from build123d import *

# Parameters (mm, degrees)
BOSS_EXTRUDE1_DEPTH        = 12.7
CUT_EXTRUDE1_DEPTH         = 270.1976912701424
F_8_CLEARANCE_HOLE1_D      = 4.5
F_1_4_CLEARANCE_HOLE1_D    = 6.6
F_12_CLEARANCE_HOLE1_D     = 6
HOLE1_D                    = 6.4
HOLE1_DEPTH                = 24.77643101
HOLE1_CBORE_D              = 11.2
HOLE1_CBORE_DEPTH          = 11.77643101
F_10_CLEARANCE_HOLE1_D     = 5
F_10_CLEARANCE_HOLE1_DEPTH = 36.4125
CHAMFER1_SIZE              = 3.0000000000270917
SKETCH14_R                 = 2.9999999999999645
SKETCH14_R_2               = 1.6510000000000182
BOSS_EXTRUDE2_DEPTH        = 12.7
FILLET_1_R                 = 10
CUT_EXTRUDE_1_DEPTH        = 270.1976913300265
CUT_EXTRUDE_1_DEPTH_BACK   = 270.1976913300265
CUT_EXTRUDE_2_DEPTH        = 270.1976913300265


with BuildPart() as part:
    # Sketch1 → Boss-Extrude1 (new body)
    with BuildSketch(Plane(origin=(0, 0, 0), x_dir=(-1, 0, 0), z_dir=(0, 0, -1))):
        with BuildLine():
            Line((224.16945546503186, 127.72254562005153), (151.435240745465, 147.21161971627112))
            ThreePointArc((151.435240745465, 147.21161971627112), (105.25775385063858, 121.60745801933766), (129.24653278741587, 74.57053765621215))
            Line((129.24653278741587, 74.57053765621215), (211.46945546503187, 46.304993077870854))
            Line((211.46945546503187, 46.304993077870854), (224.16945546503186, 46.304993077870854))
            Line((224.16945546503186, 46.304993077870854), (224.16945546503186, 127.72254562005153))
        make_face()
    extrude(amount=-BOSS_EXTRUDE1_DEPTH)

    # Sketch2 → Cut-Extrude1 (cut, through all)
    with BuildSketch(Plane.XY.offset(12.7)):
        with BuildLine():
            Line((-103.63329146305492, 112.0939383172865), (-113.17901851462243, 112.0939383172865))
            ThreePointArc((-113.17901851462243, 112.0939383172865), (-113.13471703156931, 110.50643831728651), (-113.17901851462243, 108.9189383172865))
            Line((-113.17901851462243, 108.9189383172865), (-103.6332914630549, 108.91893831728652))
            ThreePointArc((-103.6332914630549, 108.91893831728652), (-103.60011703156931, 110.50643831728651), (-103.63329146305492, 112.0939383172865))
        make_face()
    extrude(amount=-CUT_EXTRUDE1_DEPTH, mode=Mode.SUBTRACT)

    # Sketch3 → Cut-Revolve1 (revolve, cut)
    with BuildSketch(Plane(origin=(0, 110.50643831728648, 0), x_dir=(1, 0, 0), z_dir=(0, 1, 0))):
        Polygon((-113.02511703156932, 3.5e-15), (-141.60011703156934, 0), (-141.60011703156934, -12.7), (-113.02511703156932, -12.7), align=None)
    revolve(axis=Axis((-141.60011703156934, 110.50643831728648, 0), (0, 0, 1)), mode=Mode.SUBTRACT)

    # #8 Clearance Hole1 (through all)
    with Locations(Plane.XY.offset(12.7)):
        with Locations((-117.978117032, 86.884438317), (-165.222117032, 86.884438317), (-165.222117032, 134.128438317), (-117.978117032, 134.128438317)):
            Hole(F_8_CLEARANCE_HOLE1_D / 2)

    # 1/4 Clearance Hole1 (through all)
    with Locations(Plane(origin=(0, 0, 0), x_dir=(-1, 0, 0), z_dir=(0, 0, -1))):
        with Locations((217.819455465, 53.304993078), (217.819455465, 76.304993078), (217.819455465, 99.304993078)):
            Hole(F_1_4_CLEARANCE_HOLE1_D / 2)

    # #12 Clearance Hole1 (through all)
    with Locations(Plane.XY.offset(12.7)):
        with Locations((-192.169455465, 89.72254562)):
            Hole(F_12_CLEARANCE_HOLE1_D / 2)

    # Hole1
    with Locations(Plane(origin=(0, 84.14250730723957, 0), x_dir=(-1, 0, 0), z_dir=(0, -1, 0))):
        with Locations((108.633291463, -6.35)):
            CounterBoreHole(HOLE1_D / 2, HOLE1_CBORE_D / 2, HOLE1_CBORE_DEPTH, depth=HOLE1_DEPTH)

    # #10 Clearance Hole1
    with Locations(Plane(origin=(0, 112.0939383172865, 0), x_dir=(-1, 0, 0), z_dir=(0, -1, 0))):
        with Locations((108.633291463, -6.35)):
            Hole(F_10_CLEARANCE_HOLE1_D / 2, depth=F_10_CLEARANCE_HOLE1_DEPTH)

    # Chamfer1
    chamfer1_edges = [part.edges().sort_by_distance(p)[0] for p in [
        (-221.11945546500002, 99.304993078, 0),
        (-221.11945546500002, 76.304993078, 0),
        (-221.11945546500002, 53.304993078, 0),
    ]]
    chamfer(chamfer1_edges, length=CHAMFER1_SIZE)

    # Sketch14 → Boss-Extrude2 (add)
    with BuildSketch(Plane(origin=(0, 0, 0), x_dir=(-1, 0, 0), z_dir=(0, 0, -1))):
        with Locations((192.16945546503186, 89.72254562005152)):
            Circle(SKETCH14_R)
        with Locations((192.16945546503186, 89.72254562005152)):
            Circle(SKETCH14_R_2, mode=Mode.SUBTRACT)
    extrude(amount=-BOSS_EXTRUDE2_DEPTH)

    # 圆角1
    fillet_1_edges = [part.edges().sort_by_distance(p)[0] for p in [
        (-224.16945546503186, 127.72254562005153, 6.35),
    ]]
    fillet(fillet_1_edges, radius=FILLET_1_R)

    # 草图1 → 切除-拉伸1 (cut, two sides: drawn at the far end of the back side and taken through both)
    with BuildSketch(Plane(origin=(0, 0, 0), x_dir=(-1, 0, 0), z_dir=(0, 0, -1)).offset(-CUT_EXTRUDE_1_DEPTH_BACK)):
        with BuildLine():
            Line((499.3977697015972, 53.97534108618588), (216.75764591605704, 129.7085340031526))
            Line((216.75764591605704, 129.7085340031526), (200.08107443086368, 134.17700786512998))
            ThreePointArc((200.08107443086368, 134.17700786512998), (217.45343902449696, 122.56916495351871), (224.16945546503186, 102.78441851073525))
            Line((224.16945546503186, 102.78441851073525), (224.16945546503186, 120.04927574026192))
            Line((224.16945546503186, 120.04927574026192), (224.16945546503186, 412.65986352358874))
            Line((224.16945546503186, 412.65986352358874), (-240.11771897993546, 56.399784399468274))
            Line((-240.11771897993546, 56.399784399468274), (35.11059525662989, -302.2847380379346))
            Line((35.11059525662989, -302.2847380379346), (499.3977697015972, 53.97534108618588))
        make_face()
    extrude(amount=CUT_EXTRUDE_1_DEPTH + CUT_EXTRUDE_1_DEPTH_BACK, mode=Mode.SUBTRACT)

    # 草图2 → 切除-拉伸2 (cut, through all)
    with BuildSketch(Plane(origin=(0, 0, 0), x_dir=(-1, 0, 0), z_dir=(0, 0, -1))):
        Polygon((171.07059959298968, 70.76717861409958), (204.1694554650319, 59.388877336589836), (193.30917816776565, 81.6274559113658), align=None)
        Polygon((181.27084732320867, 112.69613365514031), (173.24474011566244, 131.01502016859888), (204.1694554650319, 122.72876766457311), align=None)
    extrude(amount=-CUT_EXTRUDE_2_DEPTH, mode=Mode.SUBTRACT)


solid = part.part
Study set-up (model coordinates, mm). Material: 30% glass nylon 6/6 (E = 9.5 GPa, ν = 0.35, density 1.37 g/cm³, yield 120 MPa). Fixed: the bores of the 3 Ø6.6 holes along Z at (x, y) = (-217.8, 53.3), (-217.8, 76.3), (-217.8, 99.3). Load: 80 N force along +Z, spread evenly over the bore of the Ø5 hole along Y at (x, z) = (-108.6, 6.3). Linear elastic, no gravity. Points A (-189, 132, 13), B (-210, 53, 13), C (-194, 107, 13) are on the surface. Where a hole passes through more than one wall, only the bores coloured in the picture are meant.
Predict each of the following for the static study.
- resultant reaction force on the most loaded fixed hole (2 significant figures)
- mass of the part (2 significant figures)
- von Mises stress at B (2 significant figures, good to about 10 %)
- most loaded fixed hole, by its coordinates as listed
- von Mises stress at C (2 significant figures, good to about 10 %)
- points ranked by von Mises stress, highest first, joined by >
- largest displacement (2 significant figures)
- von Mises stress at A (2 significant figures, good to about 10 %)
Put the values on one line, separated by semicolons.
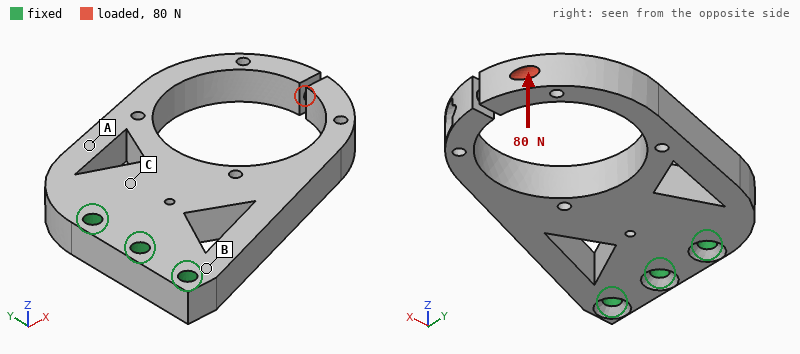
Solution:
97 N; 96 g; 2.7 MPa; (-217.8, 99.3); 5.8 MPa; A > C > B; 1.7 mm; 9.3 MPa
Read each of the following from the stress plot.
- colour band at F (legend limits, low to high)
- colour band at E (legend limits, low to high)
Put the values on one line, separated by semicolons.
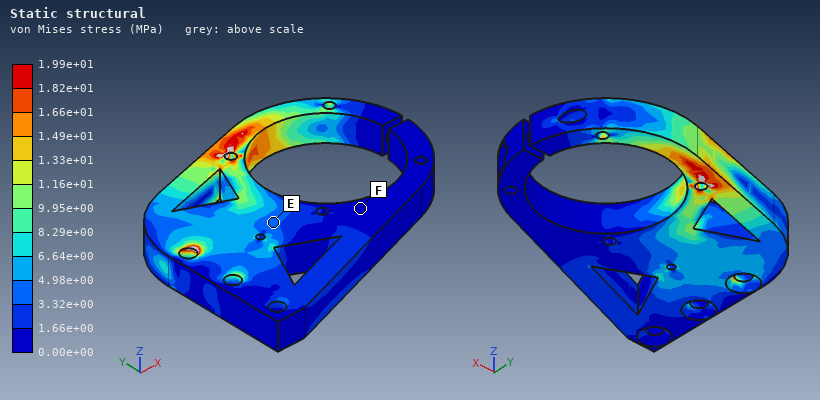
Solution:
0.00e+00 to 1.66e+00 MPa; 3.32e+00 to 4.98e+00 MPa
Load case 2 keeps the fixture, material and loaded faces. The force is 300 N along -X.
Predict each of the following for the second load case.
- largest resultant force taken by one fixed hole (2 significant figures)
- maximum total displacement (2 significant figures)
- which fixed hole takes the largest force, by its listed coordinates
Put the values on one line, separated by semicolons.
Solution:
430 N; 1.8 mm; (-217.8, 99.3)
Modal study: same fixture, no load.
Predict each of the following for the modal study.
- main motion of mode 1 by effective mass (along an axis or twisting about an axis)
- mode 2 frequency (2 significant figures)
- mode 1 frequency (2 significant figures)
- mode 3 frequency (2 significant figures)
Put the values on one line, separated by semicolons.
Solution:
along Z; 770 Hz; 480 Hz; 770 Hz
